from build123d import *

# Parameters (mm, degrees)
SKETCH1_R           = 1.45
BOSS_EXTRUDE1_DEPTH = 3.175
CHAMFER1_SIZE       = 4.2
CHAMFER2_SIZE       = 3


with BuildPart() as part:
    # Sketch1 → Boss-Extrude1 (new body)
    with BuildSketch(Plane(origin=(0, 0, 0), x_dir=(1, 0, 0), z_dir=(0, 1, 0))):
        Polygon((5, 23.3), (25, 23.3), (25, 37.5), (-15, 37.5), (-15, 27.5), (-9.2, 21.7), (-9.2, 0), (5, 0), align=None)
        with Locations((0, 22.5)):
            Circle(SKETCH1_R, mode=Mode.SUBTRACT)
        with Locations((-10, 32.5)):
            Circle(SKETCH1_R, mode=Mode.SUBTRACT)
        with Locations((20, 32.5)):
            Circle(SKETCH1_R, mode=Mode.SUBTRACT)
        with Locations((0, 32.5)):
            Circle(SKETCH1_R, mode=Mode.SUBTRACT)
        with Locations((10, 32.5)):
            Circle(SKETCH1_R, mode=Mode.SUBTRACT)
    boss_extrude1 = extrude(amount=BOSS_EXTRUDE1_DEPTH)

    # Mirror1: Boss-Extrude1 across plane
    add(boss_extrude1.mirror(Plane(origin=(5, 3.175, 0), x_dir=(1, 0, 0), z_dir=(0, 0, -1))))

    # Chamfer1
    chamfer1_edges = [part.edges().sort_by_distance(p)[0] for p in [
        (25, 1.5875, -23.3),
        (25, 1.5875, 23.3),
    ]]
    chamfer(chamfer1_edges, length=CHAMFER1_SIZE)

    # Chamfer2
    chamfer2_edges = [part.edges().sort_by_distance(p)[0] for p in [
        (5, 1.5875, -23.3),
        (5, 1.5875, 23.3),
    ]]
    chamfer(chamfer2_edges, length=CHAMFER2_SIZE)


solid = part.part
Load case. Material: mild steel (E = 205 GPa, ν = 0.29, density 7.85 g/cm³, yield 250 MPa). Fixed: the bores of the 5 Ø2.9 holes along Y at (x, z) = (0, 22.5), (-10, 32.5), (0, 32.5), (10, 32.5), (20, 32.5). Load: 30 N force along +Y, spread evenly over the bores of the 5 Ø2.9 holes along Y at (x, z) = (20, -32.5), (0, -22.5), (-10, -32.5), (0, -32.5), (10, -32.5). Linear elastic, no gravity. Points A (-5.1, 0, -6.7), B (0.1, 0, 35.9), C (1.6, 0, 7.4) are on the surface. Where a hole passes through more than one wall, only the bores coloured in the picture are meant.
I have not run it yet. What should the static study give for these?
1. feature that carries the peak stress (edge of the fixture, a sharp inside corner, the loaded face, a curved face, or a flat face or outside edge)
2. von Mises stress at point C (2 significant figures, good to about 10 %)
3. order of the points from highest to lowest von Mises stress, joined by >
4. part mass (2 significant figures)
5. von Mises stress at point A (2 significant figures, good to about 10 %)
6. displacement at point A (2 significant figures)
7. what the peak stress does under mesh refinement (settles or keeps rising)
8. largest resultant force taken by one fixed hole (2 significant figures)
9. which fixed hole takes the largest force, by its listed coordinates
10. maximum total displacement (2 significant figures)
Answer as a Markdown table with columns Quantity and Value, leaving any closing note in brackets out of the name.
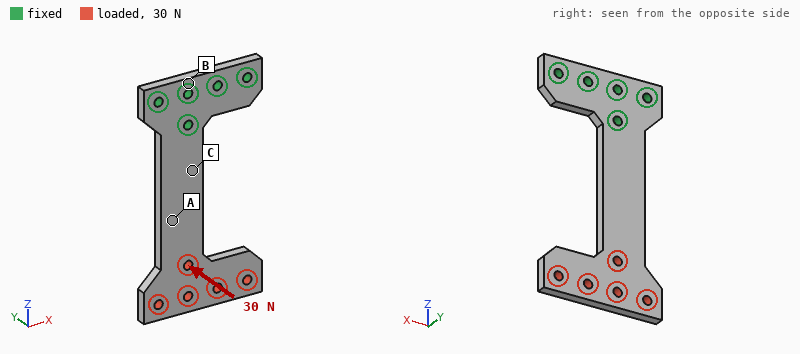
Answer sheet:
| Quantity | Value |
|---|---|
| feature that carries the peak stress | edge of the fixture |
| von Mises stress at point C | 48 MPa |
| order of the points from highest to lowest von Mises stress, joined by > | C > A > B |
| part mass | 43 g |
| von Mises stress at point A | 30 MPa |
| displacement at point A | 0.069 mm |
| what the peak stress does under mesh refinement | keeps rising |
| largest resultant force taken by one fixed hole | 100 N |
| which fixed hole takes the largest force, by its listed coordinates | (0, 22.5) |
| maximum total displacement | 0.25 mm |
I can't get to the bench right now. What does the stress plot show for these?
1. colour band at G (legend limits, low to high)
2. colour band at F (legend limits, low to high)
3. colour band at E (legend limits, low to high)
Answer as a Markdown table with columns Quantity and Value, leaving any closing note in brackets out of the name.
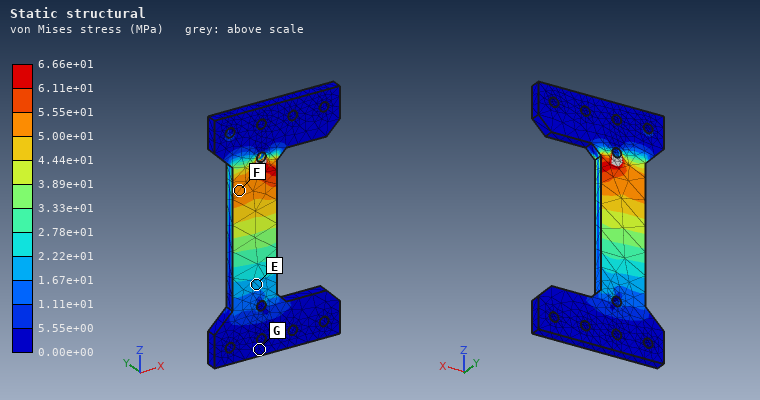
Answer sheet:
| Quantity | Value |
|---|---|
| colour band at G | 0.00e+00 to 5.55e+00 MPa |
| colour band at F | 5.00e+01 to 5.55e+01 MPa |
| colour band at E | 1.67e+01 to 2.22e+01 MPa |
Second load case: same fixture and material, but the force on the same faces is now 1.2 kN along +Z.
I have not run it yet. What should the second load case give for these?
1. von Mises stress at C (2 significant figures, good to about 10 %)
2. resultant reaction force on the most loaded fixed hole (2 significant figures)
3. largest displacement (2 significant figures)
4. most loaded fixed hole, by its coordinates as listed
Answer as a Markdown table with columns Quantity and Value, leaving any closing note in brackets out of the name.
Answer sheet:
| Quantity | Value |
|---|---|
| von Mises stress at C | 62 MPa |
| resultant reaction force on the most loaded fixed hole | 1.1 kN |
| largest displacement | 0.12 mm |
| most loaded fixed hole, by its coordinates as listed | (0, 22.5) |
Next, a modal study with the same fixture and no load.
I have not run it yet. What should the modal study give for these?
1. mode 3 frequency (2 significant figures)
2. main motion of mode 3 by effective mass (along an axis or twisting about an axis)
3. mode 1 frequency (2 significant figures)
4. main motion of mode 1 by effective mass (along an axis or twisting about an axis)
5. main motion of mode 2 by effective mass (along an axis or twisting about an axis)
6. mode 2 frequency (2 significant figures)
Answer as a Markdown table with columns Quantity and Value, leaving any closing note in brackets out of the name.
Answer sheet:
| Quantity | Value |
|---|---|
| mode 3 frequency | 1900 Hz |
| main motion of mode 3 by effective mass | along X |
| mode 1 frequency | 500 Hz |
| main motion of mode 1 by effective mass | along Y |
| main motion of mode 2 by effective mass | twisting about Z |
| mode 2 frequency | 1700 Hz |
